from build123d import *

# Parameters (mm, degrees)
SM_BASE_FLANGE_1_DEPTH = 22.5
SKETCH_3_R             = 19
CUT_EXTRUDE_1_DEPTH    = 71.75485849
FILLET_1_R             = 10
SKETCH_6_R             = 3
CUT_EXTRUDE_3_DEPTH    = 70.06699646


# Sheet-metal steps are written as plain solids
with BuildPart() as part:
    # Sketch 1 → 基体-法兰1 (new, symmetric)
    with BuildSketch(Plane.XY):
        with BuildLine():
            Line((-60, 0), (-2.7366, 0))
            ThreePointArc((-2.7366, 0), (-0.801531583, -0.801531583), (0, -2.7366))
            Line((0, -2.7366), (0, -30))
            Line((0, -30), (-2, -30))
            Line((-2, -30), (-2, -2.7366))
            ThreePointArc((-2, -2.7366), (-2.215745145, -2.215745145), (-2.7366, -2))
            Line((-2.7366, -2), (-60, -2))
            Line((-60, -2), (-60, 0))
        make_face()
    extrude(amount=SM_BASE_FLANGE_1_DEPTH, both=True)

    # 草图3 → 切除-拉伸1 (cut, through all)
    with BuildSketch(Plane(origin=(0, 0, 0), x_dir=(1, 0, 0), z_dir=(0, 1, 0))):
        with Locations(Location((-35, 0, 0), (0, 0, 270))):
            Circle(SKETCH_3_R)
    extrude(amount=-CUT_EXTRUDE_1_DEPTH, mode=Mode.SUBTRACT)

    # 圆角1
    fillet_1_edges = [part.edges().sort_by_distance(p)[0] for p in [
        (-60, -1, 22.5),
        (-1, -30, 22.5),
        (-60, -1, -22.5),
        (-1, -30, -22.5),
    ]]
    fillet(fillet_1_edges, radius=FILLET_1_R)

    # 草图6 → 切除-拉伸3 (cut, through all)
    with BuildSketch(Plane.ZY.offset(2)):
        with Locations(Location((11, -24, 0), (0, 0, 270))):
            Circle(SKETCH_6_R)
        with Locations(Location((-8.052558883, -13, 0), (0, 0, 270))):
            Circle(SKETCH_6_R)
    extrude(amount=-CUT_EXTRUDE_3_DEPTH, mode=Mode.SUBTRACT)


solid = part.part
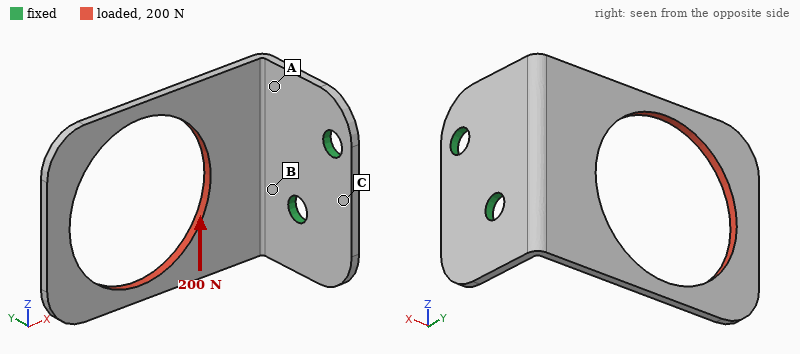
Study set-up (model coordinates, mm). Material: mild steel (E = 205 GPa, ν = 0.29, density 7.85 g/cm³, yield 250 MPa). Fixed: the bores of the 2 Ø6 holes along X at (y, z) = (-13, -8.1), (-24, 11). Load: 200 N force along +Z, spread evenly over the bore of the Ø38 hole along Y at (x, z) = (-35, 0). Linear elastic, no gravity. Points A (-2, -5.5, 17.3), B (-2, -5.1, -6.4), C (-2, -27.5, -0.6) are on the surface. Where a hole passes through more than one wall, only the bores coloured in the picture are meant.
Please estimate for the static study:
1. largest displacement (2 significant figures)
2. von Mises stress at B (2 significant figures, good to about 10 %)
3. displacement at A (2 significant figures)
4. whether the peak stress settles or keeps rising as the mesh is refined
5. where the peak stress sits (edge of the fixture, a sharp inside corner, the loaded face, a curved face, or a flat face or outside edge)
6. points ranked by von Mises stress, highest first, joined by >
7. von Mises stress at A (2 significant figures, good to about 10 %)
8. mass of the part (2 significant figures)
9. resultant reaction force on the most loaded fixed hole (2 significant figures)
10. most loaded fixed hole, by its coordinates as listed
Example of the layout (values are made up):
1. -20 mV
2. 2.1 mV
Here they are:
1. 0.37 mm
2. 140 MPa
3. 0.088 mm
4. keeps rising
5. edge of the fixture
6. B > A > C
7. 59 MPa
8. 42 g
9. 260 N
10. (-13, -8.1)
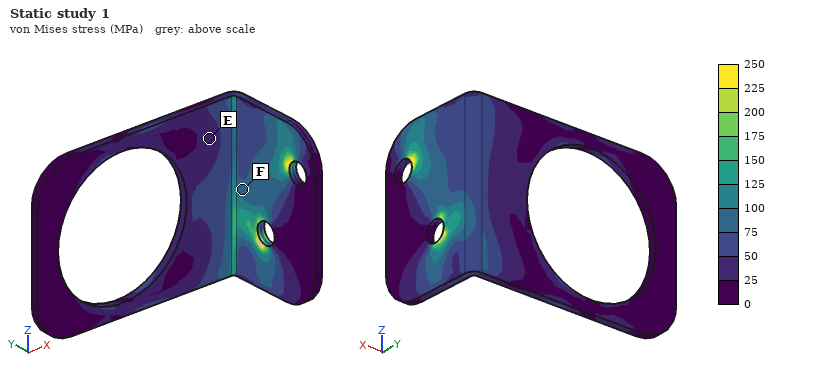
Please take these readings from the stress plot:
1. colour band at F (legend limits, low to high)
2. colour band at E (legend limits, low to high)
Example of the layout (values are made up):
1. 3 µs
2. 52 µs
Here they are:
1. 75 to 100 MPa
2. 25 to 50 MPa
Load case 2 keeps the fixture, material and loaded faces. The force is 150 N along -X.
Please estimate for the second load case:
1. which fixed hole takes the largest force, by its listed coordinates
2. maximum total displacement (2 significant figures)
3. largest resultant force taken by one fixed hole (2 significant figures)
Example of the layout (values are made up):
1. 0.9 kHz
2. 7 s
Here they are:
1. (-13, -8.1)
2. 0.14 mm
3. 130 N
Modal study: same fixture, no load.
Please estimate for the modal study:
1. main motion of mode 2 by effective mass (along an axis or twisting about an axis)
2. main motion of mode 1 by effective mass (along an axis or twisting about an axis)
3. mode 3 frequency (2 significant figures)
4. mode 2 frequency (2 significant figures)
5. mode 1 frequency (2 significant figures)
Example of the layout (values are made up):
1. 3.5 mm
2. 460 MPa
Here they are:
1. along Z
2. along Y
3. 1200 Hz
4. 980 Hz
5. 390 Hz
